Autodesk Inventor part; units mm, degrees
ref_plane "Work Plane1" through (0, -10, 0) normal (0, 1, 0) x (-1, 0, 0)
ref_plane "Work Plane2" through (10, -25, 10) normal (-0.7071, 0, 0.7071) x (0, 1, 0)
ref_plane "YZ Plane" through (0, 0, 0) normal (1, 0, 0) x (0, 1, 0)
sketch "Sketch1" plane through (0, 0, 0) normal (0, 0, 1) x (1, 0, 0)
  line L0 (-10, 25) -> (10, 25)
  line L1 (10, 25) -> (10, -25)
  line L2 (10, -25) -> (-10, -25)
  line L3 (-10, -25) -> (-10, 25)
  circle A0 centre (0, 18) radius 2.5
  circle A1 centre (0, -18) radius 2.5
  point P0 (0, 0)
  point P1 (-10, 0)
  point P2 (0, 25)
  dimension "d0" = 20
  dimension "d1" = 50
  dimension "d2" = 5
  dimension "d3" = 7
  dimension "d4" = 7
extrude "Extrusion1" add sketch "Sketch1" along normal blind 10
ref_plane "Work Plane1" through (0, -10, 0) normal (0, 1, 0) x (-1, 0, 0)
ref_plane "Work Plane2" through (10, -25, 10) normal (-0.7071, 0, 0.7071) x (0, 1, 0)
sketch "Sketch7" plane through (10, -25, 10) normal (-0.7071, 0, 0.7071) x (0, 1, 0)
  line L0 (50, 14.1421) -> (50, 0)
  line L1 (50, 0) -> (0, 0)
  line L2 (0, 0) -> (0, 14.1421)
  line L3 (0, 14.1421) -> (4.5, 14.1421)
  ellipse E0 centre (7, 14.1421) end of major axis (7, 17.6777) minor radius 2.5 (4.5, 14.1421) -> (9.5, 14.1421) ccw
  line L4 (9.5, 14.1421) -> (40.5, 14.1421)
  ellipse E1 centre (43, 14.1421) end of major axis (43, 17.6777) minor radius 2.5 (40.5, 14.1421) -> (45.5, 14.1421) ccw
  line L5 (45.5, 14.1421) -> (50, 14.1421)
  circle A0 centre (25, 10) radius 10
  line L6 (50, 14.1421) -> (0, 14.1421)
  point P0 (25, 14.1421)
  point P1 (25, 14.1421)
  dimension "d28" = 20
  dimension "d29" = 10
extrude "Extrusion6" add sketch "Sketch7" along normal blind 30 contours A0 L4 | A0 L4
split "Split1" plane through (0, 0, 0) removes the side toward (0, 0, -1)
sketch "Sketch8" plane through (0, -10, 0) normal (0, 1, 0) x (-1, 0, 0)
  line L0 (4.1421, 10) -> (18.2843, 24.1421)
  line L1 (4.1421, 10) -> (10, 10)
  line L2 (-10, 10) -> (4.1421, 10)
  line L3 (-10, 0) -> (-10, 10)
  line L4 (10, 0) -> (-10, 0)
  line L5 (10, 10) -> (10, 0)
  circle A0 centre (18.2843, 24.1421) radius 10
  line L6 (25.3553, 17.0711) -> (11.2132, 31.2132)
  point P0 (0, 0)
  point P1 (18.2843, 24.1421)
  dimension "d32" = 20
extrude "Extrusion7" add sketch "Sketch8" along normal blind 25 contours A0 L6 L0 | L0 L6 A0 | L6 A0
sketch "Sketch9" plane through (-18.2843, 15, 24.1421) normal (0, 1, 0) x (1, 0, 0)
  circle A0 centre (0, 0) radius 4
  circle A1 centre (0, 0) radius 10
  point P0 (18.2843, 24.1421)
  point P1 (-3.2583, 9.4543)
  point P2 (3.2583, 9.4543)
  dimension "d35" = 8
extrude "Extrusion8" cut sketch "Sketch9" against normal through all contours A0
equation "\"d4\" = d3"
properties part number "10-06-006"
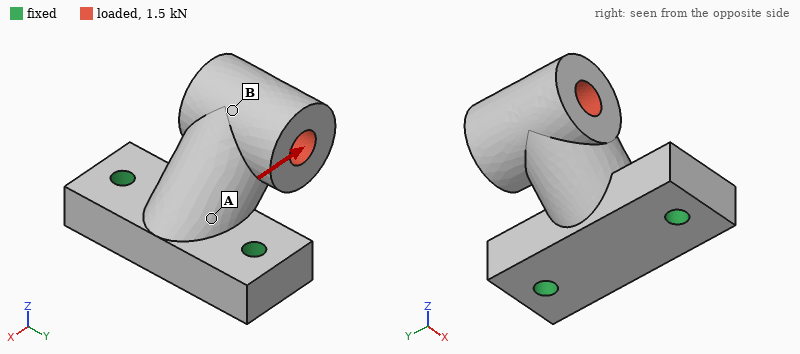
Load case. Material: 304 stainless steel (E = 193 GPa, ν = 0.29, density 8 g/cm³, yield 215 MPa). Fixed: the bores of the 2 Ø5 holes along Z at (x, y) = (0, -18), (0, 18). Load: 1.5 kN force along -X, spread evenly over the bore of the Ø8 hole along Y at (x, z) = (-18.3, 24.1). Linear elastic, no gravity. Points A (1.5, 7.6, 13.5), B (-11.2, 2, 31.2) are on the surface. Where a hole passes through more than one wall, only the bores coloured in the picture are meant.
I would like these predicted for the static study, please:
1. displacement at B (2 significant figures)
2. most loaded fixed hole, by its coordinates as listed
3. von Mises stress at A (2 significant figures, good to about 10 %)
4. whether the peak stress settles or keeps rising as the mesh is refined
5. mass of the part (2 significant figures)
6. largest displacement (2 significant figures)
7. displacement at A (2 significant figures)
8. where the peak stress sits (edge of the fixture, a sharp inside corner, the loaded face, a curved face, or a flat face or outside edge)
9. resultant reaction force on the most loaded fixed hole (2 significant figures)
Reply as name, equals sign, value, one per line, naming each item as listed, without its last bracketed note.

displacement at B = 20 µm
most loaded fixed hole, by its coordinates as listed = (0, 18)
von Mises stress at A = 27 MPa
whether the peak stress settles or keeps rising as the mesh is refined = keeps rising
mass of the part = 160 g
largest displacement = 25 µm
displacement at A = 5.5 µm
where the peak stress sits = edge of the fixture
resultant reaction force on the most loaded fixed hole = 860 N
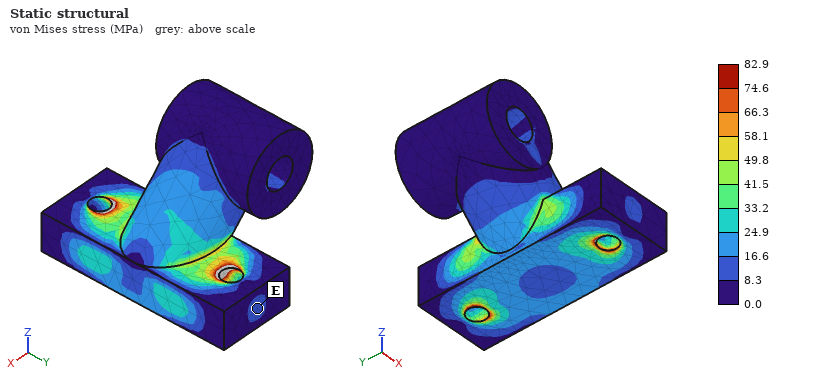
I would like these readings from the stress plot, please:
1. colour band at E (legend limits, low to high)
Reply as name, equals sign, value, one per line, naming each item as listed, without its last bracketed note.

colour band at E = 8.3 to 16.6 MPa
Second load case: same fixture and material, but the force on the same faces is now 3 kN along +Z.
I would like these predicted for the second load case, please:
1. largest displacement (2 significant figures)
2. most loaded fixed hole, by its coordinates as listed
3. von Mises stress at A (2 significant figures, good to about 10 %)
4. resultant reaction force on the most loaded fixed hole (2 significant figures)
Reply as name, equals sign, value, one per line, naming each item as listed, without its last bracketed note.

largest displacement = 48 µm
most loaded fixed hole, by its coordinates as listed = (0, 18)
von Mises stress at A = 33 MPa
resultant reaction force on the most loaded fixed hole = 1.8 kN
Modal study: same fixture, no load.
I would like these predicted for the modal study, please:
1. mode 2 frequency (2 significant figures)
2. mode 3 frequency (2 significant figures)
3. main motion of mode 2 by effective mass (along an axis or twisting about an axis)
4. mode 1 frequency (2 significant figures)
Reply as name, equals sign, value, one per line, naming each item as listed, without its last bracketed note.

mode 2 frequency = 8700 Hz
mode 3 frequency = 16 kHz
main motion of mode 2 by effective mass = along Y
mode 1 frequency = 4900 Hz
